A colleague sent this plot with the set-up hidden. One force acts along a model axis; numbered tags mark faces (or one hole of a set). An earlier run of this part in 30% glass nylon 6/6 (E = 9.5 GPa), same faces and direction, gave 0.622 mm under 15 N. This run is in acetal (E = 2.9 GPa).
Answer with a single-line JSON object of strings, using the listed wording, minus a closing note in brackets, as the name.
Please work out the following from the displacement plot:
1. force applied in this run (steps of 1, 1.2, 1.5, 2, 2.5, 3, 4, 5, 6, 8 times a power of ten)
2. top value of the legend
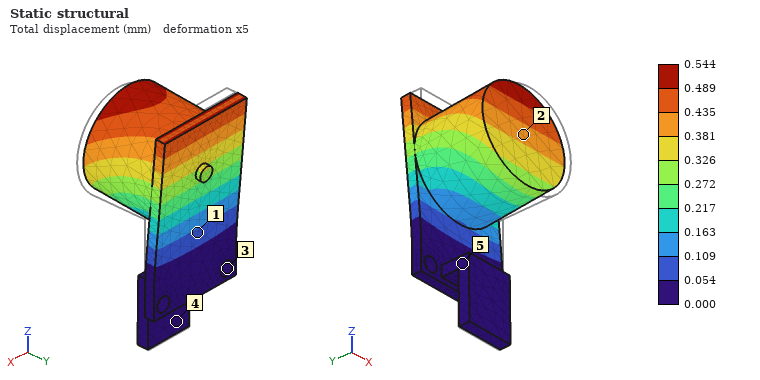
{"force applied in this run": "4 N", "top value of the legend": "0.544 mm"}
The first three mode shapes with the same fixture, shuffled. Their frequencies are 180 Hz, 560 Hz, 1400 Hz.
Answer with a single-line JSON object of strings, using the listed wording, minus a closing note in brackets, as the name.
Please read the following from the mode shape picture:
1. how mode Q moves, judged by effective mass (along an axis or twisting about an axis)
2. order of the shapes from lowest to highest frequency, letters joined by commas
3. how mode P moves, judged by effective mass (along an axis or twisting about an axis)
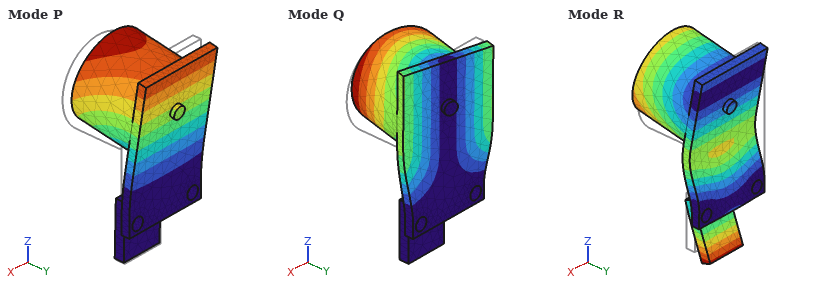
{"how mode Q moves, judged by effective mass": "along X", "order of the shapes from lowest to highest frequency, letters joined by commas": "P, Q, R", "how mode P moves, judged by effective mass": "along Y"}
